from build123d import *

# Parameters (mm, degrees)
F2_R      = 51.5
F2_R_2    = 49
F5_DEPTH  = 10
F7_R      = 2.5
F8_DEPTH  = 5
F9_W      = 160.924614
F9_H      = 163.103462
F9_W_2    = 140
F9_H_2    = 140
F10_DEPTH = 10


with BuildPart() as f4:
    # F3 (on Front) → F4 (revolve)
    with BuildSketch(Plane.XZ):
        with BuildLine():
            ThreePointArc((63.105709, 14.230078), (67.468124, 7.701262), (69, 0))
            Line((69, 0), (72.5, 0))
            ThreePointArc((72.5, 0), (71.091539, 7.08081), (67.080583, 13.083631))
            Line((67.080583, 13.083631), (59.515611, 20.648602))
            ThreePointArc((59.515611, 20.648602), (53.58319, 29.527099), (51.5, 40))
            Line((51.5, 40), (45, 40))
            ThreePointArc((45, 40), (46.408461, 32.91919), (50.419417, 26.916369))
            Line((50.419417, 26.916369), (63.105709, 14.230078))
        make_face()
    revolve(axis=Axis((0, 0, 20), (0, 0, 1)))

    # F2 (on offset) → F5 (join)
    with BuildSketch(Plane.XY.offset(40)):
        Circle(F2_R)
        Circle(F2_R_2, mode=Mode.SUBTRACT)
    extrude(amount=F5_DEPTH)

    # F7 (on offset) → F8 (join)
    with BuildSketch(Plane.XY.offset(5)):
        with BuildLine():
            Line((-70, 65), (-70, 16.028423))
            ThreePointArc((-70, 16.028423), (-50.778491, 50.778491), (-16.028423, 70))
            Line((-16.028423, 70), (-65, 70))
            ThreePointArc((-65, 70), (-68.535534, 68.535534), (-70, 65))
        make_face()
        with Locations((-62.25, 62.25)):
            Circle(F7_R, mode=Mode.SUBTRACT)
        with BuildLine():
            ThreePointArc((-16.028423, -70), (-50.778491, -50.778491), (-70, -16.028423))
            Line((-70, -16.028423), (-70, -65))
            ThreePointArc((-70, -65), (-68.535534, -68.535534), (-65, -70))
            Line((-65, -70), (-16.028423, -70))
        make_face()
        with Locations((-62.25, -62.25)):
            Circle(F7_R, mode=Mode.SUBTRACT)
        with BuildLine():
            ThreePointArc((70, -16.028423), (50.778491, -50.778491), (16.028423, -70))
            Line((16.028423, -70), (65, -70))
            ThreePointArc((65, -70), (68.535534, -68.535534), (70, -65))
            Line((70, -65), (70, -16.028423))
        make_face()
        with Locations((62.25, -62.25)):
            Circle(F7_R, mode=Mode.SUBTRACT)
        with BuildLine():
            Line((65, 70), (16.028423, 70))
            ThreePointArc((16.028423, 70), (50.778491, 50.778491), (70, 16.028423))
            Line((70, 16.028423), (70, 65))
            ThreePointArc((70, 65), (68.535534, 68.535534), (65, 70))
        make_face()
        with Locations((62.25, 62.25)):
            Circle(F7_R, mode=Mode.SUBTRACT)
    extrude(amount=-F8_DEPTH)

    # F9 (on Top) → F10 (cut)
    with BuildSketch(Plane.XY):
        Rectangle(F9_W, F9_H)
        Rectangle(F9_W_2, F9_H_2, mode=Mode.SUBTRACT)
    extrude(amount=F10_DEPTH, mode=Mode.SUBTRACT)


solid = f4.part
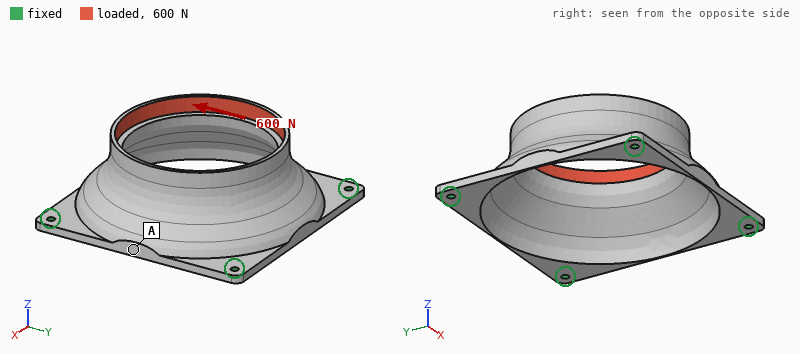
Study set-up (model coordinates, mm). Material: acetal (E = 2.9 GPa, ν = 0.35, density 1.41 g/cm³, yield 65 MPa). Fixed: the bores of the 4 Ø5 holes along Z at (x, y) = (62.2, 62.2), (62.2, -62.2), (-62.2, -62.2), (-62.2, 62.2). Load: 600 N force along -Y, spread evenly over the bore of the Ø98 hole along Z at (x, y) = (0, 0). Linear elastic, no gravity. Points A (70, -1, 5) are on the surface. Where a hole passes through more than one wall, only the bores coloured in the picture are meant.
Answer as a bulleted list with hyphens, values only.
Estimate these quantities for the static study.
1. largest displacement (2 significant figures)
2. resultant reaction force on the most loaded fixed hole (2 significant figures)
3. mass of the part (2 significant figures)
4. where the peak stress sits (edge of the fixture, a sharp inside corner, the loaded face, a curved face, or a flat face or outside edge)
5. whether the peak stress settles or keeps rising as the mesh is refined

- 0.30 mm
- 200 N
- 120 g
- edge of the fixture
- keeps rising
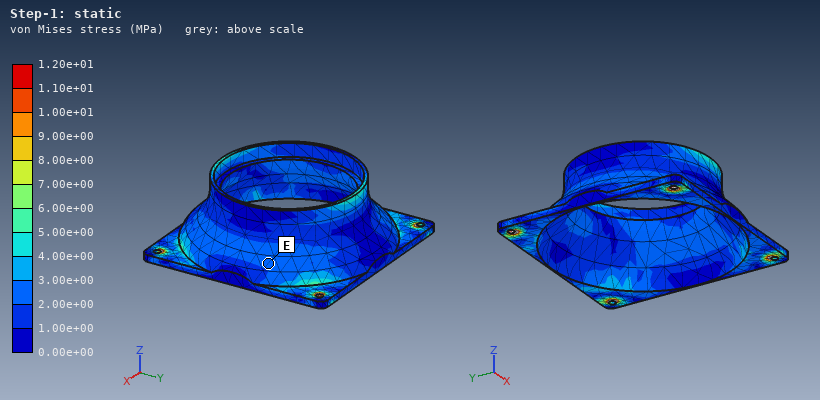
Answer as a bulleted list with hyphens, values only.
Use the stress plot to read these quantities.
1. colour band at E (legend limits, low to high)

- 2.00e+00 to 3.00e+00 MPa
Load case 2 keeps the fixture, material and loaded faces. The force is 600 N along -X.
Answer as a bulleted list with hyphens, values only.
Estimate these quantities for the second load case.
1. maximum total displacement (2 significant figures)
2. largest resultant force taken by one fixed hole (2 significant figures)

- 0.30 mm
- 200 N
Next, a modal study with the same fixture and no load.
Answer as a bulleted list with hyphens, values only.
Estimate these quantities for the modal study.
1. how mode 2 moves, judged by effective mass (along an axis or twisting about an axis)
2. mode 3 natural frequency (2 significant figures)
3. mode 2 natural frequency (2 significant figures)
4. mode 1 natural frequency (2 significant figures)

- along Z
- 910 Hz
- 850 Hz
- 650 Hz
